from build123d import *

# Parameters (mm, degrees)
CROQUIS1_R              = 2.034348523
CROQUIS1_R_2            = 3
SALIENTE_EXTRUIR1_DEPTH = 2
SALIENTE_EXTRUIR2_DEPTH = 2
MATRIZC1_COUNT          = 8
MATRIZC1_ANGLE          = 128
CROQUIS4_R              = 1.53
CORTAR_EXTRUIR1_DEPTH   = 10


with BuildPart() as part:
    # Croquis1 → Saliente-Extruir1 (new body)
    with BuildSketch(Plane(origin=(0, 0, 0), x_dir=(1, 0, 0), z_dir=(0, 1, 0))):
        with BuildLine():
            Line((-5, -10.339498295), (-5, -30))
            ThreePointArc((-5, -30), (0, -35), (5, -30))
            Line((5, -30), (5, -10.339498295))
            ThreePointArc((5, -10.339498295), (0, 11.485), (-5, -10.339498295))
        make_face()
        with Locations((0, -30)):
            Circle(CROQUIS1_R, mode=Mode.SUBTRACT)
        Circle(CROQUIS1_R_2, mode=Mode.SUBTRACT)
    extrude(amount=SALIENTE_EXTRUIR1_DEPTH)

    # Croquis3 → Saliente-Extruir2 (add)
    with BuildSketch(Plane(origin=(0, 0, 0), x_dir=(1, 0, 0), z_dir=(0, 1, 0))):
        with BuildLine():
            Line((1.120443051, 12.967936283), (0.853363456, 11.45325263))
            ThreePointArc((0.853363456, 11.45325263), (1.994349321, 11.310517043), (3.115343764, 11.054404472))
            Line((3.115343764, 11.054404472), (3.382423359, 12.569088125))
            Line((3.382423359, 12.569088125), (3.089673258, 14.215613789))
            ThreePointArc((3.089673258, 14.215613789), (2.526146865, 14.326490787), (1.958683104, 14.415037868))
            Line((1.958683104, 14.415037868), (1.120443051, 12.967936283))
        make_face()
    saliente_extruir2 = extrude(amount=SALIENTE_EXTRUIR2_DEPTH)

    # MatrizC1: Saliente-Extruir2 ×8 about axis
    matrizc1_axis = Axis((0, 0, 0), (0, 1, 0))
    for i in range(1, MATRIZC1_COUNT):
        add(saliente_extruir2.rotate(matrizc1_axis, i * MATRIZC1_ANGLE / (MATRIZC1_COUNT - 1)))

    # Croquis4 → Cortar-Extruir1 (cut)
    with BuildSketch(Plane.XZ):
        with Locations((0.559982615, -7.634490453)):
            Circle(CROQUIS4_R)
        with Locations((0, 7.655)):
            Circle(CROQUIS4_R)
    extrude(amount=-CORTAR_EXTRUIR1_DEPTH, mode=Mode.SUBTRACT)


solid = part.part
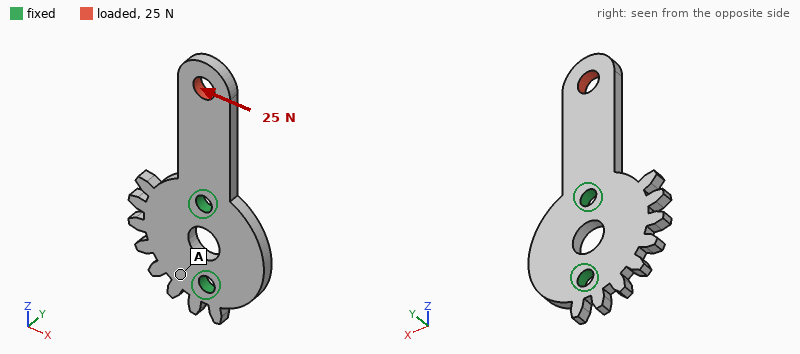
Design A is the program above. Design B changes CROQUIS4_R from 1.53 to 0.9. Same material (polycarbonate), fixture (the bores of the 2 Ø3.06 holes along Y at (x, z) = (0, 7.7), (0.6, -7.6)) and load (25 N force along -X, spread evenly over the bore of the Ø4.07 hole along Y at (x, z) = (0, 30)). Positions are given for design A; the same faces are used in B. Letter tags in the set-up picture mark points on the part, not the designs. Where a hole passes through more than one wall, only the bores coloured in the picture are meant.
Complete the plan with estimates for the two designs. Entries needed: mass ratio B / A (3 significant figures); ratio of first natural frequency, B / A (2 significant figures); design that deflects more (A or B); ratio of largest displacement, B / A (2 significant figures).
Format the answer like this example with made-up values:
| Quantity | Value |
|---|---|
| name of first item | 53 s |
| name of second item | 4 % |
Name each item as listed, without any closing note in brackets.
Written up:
| Quantity | Value |
|---|---|
| mass ratio B / A | 1.02 |
| ratio of first natural frequency, B / A | 0.94 |
| design that deflects more | B |
| ratio of largest displacement, B / A | 1.1 |
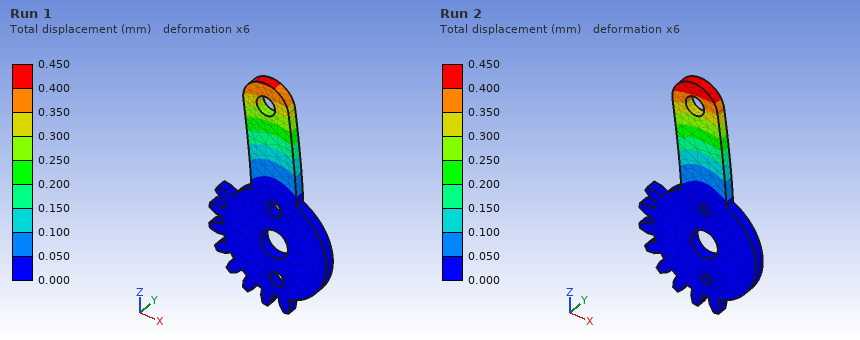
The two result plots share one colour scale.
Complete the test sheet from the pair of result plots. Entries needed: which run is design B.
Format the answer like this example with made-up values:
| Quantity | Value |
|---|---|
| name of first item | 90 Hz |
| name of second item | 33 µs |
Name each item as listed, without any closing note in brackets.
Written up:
| Quantity | Value |
|---|---|
| which run is design B | Run 2 |
